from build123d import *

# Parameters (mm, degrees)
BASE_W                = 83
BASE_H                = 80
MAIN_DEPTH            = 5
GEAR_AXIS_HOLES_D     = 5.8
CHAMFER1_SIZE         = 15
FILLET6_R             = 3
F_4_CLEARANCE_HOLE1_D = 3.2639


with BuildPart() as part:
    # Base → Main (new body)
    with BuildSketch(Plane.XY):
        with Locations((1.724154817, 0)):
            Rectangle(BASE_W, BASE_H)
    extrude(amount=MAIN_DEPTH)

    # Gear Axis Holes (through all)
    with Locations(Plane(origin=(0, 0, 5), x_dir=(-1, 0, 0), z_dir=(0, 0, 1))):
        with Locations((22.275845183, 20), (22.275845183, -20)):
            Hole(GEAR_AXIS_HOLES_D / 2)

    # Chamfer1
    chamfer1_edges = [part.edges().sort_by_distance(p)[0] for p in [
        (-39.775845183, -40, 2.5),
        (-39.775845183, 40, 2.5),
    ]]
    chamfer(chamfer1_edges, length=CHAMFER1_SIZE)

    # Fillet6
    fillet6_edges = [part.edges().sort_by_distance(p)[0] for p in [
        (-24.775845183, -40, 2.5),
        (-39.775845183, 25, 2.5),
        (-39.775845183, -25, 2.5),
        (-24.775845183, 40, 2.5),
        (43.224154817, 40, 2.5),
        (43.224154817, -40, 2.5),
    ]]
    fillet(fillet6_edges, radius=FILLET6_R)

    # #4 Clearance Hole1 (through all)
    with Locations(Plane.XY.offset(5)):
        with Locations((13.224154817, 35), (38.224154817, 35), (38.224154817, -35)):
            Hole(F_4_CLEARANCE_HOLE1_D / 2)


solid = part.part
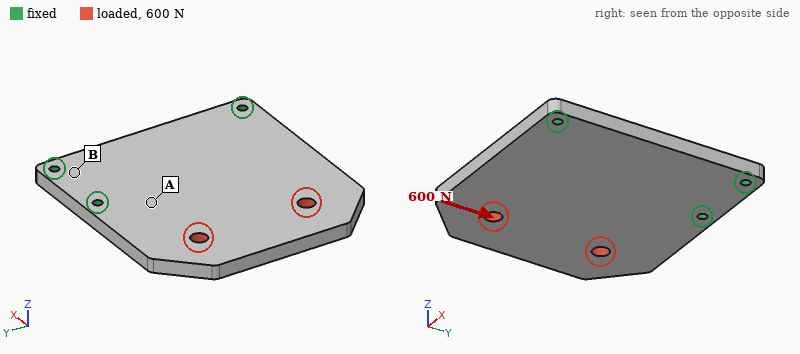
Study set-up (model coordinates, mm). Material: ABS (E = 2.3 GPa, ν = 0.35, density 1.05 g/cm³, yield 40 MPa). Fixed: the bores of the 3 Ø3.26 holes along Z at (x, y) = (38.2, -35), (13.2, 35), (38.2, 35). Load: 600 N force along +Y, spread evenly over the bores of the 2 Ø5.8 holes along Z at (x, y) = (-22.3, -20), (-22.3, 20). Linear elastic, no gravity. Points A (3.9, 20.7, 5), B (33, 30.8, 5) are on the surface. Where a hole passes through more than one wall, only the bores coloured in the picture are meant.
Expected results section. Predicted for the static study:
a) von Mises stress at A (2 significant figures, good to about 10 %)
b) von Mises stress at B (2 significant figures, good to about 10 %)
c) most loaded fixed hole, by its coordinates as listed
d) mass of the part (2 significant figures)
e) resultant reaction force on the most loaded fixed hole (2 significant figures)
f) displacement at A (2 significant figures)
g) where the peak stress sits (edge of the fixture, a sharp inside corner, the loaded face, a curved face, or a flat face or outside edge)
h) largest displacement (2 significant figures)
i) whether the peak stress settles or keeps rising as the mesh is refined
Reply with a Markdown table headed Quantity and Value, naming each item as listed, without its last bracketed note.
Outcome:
| Quantity | Value |
|---|---|
| von Mises stress at A | 4.1 MPa |
| von Mises stress at B | 1.8 MPa |
| most loaded fixed hole, by its coordinates as listed | (13.2, 35) |
| mass of the part | 33 g |
| resultant reaction force on the most loaded fixed hole | 490 N |
| displacement at A | 0.052 mm |
| where the peak stress sits | edge of the fixture |
| largest displacement | 0.19 mm |
| whether the peak stress settles or keeps rising as the mesh is refined | keeps rising |
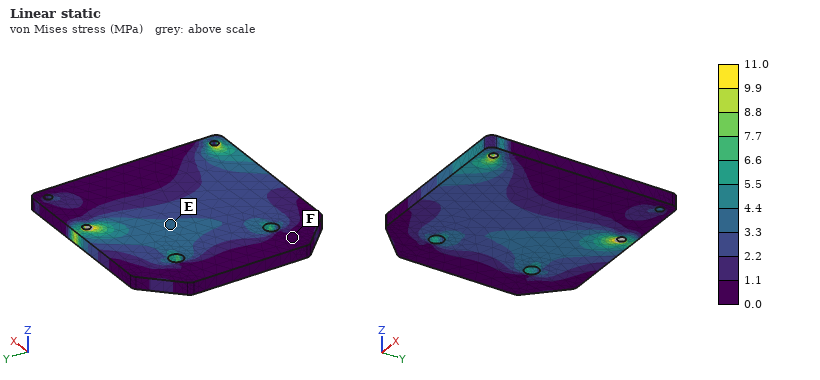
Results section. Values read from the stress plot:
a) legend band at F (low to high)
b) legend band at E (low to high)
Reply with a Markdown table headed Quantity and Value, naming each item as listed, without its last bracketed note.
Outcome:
| Quantity | Value |
|---|---|
| legend band at F | 0.0 to 1.1 MPa |
| legend band at E | 3.3 to 4.4 MPa |
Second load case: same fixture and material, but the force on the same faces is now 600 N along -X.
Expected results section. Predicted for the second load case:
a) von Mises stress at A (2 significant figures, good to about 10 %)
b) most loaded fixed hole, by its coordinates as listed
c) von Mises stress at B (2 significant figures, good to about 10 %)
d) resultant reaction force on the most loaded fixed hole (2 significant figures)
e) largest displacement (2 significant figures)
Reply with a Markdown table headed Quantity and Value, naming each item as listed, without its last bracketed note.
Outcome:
| Quantity | Value |
|---|---|
| von Mises stress at A | 1.5 MPa |
| most loaded fixed hole, by its coordinates as listed | (38.2, -35) |
| von Mises stress at B | 2.2 MPa |
| resultant reaction force on the most loaded fixed hole | 300 N |
| largest displacement | 82 µm |
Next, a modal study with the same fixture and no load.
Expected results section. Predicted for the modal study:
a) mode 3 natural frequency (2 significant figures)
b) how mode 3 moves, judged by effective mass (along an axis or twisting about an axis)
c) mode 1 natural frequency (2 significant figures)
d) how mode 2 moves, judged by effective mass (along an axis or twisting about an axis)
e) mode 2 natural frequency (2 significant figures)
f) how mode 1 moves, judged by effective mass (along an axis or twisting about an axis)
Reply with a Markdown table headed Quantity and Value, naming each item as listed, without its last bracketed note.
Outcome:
| Quantity | Value |
|---|---|
| mode 3 natural frequency | 1200 Hz |
| how mode 3 moves, judged by effective mass | along Z |
| mode 1 natural frequency | 250 Hz |
| how mode 2 moves, judged by effective mass | twisting about X |
| mode 2 natural frequency | 690 Hz |
| how mode 1 moves, judged by effective mass | along Z |
